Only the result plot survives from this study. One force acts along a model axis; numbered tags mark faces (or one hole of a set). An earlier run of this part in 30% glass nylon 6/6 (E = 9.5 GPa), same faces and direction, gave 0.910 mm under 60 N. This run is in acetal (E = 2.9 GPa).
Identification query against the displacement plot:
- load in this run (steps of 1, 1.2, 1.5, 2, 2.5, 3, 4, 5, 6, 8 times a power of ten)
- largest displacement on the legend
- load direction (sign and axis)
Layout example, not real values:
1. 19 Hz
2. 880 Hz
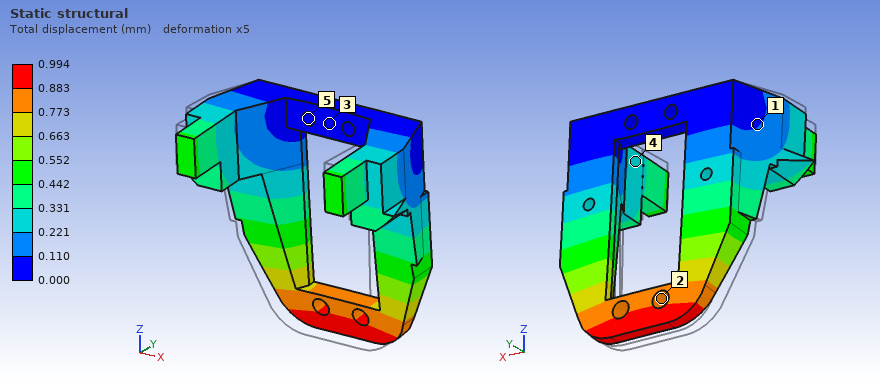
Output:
1. 20 N
2. 0.994 mm
3. +Y
